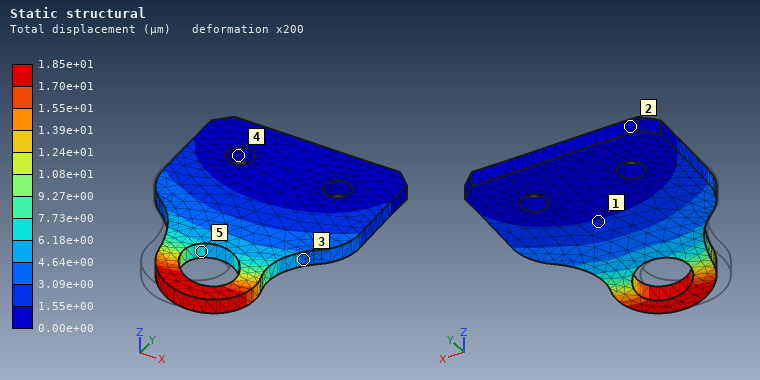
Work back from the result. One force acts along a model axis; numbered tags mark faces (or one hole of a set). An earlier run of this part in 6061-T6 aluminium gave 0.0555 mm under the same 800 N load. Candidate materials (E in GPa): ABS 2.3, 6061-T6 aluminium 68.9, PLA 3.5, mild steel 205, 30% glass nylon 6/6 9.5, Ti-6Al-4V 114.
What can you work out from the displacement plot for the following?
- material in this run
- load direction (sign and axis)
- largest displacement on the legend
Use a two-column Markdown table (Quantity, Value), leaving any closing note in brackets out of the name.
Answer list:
| Quantity | Value |
|---|---|
| material in this run | mild steel |
| load direction | +X |
| largest displacement on the legend | 1.85e+01 µm |
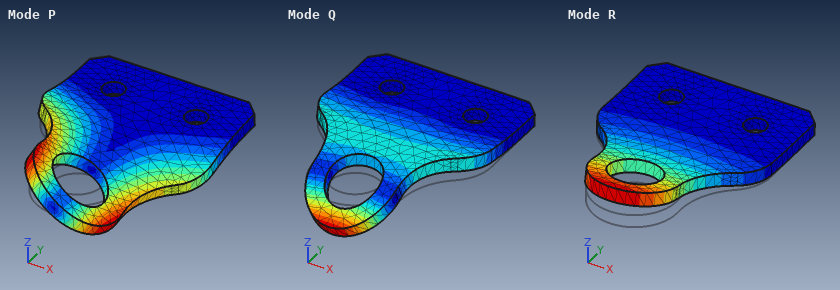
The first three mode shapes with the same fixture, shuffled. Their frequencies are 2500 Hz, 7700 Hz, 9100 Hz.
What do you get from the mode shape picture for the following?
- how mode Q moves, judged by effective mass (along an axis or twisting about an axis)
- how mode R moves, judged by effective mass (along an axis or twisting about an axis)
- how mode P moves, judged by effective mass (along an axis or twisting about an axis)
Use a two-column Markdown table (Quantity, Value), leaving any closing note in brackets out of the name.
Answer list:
| Quantity | Value |
|---|---|
| how mode Q moves, judged by effective mass | along Z |
| how mode R moves, judged by effective mass | along Z |
| how mode P moves, judged by effective mass | twisting about Y |
